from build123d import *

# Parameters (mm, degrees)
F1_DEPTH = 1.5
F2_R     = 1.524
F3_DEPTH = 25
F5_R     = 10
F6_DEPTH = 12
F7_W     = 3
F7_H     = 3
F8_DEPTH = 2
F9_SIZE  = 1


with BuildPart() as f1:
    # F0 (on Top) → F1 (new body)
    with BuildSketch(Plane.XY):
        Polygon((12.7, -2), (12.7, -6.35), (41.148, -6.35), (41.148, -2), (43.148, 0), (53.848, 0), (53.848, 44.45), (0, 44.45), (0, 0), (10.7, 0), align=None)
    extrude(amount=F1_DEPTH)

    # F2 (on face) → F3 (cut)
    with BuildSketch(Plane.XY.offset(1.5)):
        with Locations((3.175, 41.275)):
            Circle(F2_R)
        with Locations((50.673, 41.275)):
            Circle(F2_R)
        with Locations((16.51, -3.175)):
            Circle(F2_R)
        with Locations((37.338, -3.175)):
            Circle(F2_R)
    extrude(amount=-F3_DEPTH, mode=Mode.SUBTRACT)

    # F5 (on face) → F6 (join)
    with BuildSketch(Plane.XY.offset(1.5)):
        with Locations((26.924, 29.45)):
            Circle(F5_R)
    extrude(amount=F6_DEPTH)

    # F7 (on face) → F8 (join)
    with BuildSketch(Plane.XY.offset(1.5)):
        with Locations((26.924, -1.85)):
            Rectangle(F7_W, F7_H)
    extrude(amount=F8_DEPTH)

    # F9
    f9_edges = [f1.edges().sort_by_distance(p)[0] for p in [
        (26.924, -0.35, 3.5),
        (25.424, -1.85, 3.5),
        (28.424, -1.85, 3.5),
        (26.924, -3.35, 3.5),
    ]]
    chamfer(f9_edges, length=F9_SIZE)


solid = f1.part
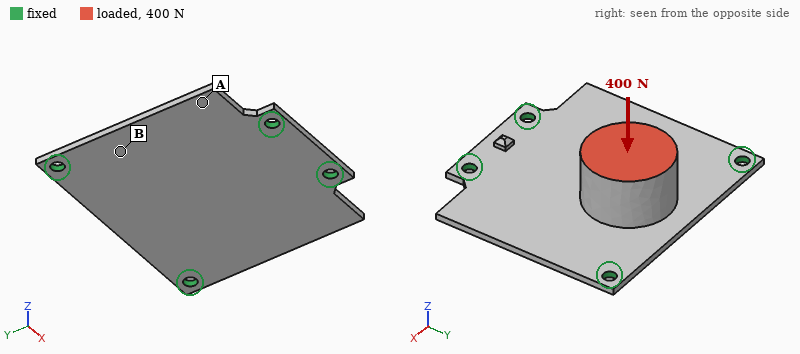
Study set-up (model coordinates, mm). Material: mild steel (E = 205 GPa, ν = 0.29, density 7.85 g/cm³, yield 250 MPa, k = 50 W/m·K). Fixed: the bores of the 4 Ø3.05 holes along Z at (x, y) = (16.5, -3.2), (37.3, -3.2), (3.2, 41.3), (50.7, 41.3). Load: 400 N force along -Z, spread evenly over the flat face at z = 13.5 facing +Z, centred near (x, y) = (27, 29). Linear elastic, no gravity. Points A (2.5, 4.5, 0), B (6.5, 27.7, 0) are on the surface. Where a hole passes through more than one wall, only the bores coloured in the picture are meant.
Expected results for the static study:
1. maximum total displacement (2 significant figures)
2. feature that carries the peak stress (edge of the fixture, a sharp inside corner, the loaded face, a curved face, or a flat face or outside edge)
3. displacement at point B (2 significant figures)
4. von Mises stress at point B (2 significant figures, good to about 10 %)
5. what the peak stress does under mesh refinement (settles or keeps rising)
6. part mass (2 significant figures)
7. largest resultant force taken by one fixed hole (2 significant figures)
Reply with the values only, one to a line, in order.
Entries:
64 µm
edge of the fixture
34 µm
47 MPa
keeps rising
60 g
160 N
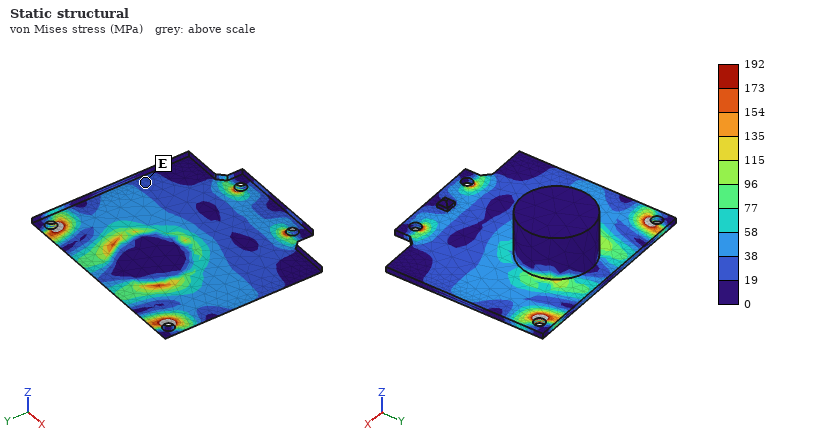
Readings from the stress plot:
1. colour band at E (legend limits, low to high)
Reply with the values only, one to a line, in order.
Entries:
19 to 38 MPa
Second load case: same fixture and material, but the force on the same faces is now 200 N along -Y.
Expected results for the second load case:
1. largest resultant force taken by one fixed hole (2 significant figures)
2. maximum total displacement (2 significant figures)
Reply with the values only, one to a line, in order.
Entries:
69 N
35 µm
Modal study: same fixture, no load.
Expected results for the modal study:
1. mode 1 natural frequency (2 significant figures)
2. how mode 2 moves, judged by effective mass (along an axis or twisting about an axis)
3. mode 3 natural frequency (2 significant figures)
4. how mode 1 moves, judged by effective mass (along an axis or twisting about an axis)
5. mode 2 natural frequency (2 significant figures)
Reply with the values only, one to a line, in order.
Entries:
1900 Hz
along Y
3200 Hz
along Z
2900 Hz
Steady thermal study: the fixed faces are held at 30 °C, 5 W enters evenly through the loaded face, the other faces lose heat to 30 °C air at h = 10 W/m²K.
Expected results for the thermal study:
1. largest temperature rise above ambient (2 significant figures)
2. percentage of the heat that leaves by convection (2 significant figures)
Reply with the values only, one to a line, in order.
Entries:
24 K
14 %
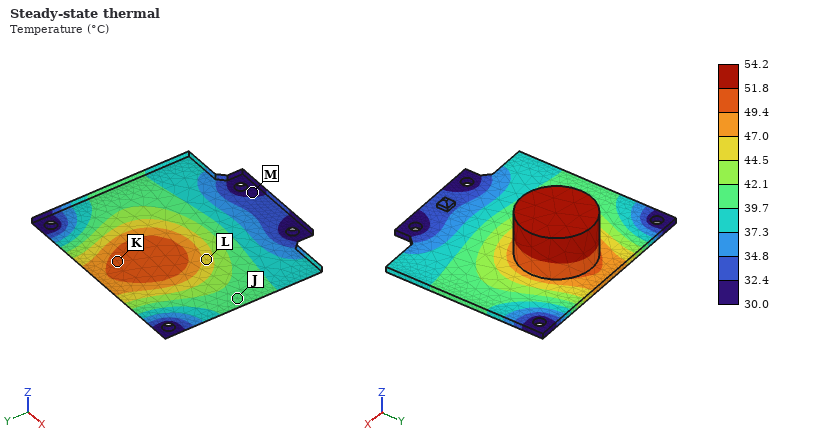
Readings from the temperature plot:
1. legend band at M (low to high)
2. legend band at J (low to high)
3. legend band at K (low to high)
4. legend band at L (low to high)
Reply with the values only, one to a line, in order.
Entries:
30.0 to 32.4 °C
39.7 to 42.1 °C
49.4 to 51.8 °C
44.5 to 47.0 °C
